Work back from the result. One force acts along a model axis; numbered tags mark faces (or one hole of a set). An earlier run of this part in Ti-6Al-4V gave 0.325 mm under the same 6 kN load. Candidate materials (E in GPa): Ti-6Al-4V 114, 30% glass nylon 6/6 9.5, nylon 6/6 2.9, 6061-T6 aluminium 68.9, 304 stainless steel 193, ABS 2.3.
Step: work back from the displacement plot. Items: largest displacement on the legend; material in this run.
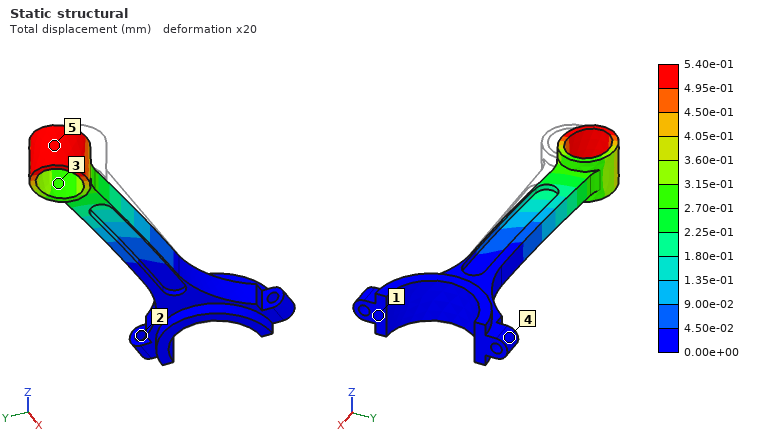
5.40e-01 mm
6061-T6 aluminium
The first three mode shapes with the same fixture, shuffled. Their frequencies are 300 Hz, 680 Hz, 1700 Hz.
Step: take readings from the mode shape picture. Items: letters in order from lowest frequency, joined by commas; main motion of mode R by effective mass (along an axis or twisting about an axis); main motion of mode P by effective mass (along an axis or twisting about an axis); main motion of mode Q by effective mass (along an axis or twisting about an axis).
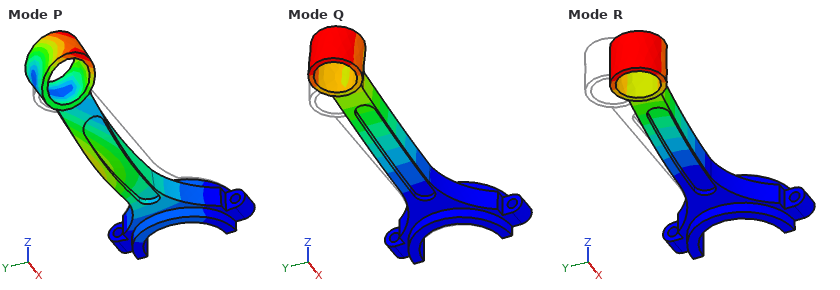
Q, R, P
along Y
along Z
along Z
